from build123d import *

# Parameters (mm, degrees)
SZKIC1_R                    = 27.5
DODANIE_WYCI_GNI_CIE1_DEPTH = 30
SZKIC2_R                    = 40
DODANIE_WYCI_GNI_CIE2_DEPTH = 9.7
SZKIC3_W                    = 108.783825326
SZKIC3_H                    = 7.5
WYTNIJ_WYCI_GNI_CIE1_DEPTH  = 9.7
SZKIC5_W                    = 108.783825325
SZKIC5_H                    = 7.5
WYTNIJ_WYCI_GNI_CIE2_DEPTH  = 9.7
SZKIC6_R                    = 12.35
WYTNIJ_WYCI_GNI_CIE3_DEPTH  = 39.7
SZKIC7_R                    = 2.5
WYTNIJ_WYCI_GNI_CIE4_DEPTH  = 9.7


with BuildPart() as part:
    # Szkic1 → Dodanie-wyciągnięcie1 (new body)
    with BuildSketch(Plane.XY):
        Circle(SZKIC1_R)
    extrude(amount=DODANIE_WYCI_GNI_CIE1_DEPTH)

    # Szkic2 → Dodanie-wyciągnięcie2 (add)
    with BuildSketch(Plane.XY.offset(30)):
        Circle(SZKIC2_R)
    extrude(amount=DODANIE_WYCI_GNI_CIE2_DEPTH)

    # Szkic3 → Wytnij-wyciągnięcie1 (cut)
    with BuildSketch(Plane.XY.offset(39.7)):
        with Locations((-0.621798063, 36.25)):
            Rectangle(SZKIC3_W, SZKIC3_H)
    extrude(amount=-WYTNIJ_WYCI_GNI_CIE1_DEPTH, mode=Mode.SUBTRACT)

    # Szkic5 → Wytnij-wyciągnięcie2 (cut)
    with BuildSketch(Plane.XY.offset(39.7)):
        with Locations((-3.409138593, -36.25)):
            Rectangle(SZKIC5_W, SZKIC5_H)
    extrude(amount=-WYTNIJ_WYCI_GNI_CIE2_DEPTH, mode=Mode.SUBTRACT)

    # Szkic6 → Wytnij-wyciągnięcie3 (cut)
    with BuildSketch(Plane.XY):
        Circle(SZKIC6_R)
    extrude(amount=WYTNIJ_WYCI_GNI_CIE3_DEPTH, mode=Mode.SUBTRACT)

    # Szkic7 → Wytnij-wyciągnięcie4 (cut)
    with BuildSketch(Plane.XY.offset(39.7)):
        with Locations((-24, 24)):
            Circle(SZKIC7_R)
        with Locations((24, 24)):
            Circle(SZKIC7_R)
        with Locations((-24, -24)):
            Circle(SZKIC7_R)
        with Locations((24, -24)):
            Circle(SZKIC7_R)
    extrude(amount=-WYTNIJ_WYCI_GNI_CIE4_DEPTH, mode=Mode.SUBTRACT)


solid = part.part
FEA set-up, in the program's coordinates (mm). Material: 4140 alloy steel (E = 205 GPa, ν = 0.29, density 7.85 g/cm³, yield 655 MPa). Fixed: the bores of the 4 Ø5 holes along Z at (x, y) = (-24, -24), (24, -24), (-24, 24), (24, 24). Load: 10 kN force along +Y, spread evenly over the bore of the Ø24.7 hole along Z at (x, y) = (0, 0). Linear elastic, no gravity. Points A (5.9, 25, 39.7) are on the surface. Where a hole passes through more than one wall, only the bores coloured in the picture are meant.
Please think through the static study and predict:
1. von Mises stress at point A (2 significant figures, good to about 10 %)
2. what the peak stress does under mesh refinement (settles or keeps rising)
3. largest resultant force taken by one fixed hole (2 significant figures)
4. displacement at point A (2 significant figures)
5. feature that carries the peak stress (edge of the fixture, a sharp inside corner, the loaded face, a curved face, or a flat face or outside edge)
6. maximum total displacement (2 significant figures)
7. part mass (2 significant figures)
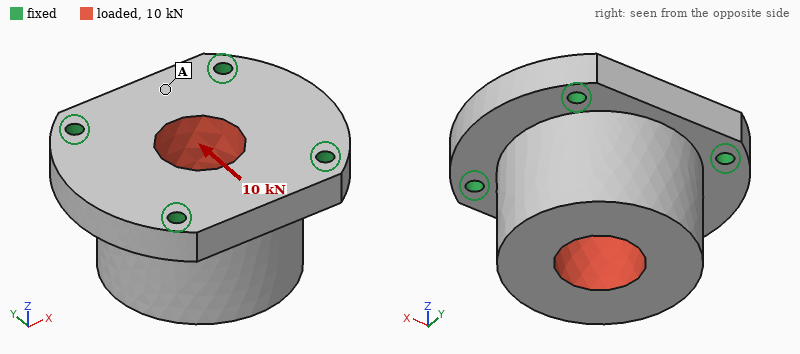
8.0 MPa
keeps rising
3.1 kN
2.2 µm
edge of the fixture
5.9 µm
750 g
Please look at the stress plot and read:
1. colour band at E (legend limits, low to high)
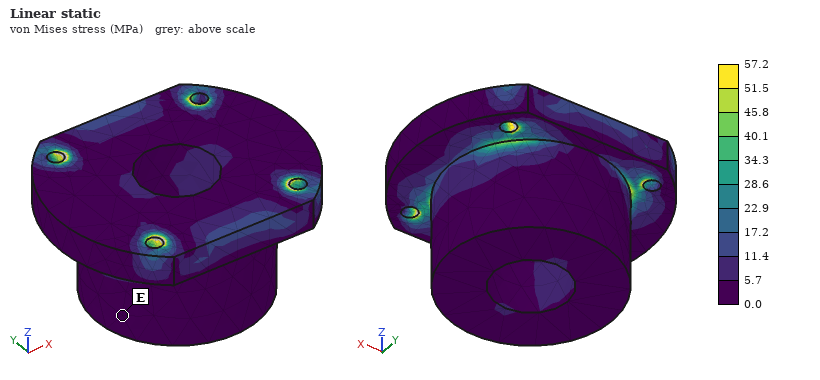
0.0 to 5.7 MPa
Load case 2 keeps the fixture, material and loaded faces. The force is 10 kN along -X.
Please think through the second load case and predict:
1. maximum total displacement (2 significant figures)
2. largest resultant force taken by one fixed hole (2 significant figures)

5.6 µm
3.0 kN
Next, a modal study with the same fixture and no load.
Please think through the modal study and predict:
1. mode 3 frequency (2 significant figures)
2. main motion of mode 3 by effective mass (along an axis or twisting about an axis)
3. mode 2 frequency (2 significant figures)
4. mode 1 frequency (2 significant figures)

11 kHz
along Z
9600 Hz
9600 Hz
